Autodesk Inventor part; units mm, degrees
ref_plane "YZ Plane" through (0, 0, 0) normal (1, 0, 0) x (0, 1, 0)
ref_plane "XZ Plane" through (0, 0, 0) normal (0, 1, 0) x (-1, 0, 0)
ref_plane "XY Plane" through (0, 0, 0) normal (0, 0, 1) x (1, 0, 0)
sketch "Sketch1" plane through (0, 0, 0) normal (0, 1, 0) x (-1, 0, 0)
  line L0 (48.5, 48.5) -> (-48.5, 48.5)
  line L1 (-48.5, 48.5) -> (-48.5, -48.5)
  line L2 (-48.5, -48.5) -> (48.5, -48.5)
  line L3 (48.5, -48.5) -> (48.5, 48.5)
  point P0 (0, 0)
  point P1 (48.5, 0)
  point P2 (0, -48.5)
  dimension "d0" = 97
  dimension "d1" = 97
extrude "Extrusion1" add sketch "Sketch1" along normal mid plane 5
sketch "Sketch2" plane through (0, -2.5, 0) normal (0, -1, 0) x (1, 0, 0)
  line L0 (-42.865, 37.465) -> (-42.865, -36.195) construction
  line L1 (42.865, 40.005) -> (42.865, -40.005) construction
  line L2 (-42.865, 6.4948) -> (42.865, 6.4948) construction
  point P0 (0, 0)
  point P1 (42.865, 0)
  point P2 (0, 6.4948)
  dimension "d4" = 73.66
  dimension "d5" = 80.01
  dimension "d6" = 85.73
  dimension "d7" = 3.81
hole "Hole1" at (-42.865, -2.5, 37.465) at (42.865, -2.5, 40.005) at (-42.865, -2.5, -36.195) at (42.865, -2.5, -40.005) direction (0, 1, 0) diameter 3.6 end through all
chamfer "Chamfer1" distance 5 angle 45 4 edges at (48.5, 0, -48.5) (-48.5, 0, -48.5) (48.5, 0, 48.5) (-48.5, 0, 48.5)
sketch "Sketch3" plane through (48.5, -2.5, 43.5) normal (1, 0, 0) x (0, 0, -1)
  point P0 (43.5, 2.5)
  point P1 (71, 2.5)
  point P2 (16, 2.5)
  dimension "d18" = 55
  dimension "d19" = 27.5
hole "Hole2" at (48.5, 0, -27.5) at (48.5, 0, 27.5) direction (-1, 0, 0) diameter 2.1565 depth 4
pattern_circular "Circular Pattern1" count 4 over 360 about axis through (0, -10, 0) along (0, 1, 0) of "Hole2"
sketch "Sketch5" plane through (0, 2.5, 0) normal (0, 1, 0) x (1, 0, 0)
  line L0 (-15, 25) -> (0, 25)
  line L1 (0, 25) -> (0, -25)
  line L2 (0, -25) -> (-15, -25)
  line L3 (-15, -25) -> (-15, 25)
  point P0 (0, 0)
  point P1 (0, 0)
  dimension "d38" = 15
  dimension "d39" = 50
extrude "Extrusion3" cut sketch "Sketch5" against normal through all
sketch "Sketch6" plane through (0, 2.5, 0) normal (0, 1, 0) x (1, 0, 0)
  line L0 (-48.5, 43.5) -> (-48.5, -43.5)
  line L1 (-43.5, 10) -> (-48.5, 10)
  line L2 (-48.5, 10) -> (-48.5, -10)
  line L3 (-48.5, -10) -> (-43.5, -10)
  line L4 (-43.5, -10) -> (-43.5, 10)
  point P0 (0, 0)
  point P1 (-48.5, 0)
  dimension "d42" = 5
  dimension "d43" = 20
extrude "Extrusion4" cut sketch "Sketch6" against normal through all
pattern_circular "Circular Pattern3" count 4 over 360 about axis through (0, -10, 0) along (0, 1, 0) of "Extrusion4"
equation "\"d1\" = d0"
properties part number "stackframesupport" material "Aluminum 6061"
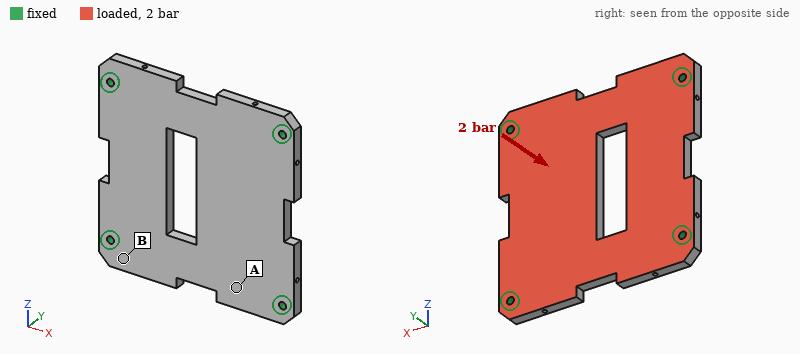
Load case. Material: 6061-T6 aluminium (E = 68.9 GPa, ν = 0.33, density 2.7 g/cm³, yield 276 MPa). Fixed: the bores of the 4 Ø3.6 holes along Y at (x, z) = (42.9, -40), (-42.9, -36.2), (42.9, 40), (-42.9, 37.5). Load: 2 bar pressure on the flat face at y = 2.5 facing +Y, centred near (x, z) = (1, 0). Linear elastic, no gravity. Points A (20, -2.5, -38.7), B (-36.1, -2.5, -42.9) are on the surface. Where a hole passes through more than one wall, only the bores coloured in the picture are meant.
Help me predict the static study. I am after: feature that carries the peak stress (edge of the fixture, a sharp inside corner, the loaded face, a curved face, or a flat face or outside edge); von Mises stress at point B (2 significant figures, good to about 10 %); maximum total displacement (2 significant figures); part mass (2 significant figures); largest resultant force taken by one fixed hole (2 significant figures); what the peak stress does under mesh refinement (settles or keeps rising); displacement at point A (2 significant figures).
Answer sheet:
edge of the fixture
23 MPa
0.13 mm
110 g
420 N
keeps rising
0.046 mm
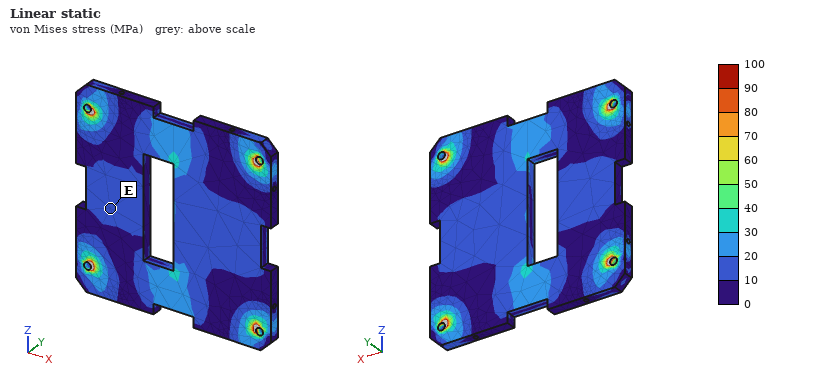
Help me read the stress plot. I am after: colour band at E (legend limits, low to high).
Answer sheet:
10 to 20 MPa
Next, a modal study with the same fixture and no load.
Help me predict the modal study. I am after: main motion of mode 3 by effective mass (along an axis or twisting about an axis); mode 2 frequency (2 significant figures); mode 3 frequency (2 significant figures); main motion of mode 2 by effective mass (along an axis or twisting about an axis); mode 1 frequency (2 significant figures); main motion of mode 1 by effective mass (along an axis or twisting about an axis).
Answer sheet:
twisting about Z
3800 Hz
4000 Hz
twisting about X
2300 Hz
along Y
